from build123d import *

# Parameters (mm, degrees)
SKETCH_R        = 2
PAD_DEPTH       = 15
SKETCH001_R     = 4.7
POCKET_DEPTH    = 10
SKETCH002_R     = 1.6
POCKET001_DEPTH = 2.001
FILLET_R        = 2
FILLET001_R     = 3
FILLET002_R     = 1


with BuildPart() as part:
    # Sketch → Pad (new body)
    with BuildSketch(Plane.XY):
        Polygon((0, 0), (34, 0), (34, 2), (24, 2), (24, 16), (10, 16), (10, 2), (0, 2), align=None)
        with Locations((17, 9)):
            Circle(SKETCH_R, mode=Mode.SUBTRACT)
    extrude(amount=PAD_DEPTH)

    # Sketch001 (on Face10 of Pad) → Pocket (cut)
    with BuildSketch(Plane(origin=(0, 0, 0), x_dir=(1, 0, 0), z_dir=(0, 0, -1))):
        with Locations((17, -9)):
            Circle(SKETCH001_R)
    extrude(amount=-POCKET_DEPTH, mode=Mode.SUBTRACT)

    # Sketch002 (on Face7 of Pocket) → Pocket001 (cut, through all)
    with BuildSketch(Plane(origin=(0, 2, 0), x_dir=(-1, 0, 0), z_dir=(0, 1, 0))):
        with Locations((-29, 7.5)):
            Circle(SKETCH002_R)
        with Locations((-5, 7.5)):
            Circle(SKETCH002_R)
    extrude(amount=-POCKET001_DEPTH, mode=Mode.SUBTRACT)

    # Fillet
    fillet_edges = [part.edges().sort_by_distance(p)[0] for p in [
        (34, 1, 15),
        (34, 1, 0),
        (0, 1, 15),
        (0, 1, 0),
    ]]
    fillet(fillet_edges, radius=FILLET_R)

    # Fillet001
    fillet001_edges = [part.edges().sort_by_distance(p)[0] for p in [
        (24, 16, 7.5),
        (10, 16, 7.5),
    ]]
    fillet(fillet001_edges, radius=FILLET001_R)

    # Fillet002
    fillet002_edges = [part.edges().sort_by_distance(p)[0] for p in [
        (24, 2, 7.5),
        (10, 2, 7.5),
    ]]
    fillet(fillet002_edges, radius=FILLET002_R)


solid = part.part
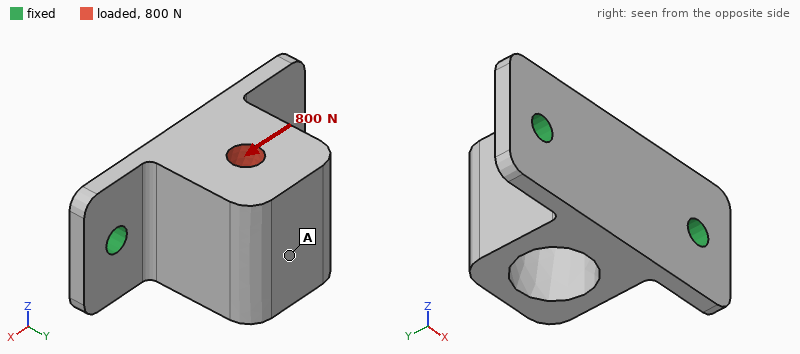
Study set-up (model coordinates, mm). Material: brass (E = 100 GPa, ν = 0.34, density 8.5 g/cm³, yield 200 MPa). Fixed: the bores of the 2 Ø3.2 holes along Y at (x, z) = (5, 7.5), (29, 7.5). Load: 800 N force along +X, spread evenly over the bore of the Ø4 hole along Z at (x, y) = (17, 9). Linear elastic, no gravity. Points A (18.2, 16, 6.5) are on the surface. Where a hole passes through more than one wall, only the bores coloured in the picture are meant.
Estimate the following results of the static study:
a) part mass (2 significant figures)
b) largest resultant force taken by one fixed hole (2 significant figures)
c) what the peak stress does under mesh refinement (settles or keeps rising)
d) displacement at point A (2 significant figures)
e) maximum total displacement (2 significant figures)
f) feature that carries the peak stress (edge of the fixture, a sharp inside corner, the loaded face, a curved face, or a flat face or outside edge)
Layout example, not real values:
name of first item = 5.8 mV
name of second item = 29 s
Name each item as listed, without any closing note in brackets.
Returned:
part mass = 26 g
largest resultant force taken by one fixed hole = 550 N
what the peak stress does under mesh refinement = keeps rising
displacement at point A = 14 µm
maximum total displacement = 16 µm
feature that carries the peak stress = edge of the fixture
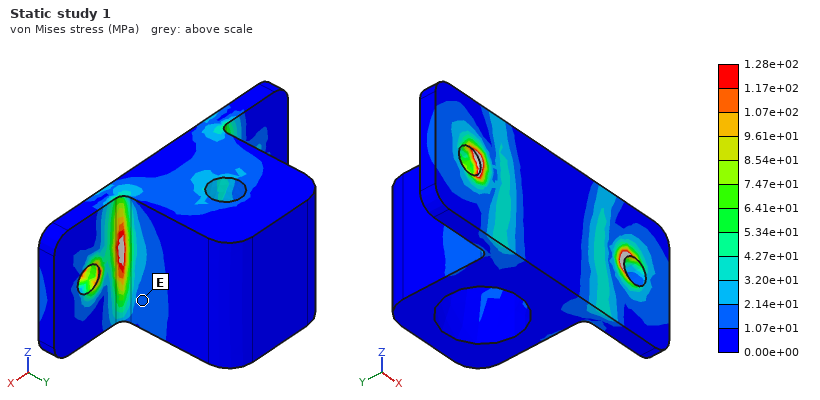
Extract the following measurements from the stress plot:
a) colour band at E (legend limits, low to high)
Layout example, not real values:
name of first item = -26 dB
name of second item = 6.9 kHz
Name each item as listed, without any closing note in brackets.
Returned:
colour band at E = 1.07e+01 to 2.14e+01 MPa
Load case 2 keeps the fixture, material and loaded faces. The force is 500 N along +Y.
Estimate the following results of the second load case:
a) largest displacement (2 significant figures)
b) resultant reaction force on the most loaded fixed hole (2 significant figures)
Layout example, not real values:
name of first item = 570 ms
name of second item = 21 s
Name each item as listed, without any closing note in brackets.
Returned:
largest displacement = 49 µm
resultant reaction force on the most loaded fixed hole = 290 N
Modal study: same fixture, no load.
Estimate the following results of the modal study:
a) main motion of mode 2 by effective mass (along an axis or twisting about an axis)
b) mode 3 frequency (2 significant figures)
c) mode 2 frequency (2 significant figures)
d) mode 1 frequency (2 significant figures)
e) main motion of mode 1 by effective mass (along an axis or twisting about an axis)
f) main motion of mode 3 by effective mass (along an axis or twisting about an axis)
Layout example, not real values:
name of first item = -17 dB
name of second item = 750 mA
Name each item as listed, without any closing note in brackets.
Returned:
main motion of mode 2 by effective mass = along X
mode 3 frequency = 9900 Hz
mode 2 frequency = 9300 Hz
mode 1 frequency = 3400 Hz
main motion of mode 1 by effective mass = along Z
main motion of mode 3 by effective mass = along Y
